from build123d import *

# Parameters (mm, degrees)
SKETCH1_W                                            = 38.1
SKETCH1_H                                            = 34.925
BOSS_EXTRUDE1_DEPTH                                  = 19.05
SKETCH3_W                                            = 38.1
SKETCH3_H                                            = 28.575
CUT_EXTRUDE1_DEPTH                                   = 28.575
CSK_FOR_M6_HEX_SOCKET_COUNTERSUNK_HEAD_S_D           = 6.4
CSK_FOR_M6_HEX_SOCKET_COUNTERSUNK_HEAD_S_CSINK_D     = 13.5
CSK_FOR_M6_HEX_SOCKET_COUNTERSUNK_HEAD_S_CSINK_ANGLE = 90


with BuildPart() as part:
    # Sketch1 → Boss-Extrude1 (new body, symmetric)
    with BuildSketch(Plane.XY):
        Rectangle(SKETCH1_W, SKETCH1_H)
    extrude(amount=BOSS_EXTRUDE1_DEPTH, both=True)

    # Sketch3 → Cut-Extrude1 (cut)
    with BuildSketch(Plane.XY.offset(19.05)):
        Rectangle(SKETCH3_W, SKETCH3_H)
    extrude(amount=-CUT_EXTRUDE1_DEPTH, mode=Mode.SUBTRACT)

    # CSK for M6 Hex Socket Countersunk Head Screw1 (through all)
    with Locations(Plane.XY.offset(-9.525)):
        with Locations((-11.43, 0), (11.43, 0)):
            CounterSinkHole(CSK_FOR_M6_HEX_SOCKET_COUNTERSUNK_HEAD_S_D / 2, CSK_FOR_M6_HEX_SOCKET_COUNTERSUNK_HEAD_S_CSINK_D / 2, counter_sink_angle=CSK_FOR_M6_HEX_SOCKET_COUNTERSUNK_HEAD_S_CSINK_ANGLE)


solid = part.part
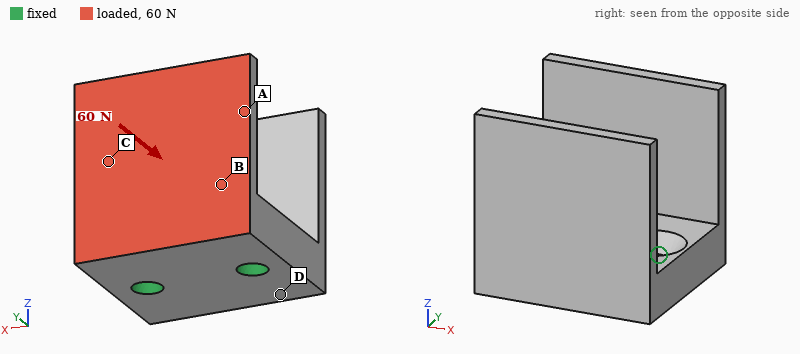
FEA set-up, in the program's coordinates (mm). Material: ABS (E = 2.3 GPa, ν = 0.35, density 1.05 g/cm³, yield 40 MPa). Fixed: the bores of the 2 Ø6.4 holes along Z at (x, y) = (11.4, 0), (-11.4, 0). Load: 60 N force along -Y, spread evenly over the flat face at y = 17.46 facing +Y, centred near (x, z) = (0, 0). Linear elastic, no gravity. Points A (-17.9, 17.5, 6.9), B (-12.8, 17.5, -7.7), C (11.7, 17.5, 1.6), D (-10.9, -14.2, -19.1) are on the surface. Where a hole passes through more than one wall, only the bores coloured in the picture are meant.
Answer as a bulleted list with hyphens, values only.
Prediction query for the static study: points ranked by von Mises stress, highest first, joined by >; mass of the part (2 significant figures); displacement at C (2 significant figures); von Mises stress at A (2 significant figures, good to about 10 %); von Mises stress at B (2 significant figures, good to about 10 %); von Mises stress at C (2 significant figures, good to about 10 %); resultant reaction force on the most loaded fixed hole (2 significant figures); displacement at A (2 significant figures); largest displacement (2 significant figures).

- B > C > A > D
- 20 g
- 0.23 mm
- 1.9 MPa
- 7.7 MPa
- 3.5 MPa
- 30 N
- 0.36 mm
- 0.75 mm
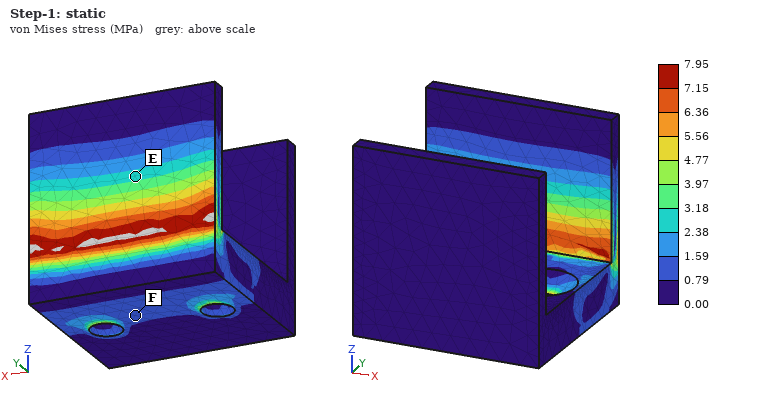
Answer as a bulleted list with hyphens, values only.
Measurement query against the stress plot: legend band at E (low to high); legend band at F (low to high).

- 2.38 to 3.18 MPa
- 0.79 to 1.59 MPa
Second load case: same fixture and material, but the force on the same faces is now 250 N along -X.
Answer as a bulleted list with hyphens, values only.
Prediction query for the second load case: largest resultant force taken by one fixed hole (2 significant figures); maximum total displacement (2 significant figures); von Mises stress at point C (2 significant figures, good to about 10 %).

- 250 N
- 0.25 mm
- 2.9 MPa
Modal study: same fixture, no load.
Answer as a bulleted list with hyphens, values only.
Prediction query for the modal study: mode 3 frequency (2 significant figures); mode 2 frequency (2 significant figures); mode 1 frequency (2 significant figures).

- 1600 Hz
- 820 Hz
- 790 Hz
